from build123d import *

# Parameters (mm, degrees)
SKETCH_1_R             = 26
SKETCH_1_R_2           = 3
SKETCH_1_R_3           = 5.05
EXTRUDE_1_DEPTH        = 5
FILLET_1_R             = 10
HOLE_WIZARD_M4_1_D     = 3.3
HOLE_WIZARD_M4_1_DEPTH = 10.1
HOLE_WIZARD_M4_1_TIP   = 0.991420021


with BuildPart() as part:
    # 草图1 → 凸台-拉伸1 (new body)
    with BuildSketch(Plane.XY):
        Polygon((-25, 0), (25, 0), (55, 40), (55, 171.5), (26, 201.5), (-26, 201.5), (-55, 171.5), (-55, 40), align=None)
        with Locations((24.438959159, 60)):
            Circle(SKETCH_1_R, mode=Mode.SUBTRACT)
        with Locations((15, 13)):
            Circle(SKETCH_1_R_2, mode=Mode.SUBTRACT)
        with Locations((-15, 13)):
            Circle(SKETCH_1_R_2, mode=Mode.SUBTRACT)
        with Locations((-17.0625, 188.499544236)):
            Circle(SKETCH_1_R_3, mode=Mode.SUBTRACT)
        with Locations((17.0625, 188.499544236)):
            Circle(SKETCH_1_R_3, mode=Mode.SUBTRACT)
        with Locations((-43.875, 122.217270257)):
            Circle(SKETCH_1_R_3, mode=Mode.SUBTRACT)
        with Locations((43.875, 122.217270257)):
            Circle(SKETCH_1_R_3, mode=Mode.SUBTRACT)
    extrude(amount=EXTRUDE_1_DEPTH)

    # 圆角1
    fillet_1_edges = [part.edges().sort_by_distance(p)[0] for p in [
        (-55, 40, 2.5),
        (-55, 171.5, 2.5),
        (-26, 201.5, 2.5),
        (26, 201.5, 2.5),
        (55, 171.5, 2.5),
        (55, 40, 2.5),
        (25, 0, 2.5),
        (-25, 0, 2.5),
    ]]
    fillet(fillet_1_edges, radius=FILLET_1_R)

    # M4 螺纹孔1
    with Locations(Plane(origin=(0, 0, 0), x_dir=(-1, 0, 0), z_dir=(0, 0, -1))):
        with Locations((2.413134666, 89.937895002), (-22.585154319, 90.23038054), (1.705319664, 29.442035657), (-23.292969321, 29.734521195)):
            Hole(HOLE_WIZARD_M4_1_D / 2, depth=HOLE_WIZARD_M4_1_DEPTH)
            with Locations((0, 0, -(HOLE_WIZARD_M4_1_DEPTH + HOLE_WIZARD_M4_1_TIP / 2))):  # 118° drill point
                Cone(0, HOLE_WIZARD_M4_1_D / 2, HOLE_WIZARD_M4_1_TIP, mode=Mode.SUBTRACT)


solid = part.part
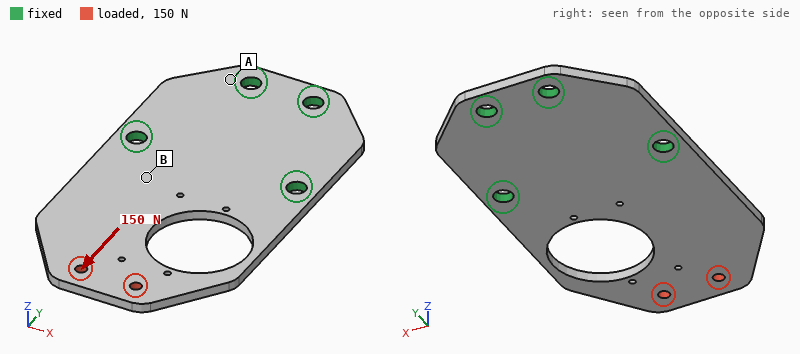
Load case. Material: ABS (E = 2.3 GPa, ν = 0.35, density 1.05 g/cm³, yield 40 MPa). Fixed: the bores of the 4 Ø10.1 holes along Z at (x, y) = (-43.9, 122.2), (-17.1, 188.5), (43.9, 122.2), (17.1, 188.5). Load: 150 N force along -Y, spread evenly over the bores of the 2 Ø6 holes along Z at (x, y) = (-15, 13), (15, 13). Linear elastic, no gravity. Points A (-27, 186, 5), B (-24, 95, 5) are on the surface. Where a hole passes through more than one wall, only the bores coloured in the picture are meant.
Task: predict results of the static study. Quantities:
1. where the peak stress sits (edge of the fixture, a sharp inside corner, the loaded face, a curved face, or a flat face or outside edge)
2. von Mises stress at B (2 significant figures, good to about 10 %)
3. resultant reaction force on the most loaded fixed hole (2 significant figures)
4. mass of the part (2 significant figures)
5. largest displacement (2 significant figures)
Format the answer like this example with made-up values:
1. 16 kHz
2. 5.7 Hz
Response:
1. a curved face
2. 0.46 MPa
3. 62 N
4. 92 g
5. 71 µm
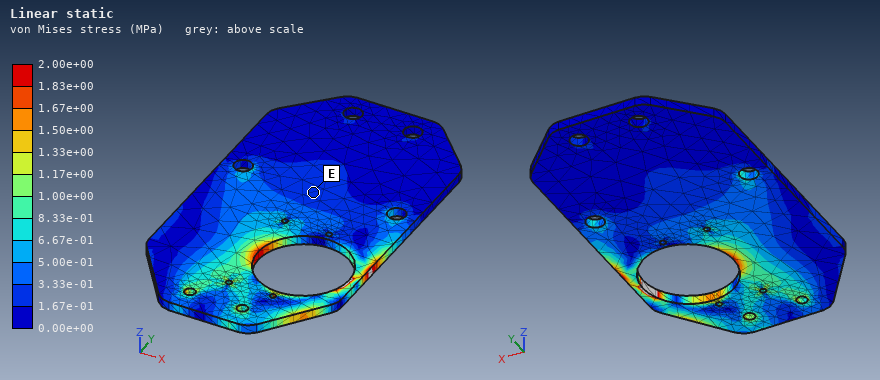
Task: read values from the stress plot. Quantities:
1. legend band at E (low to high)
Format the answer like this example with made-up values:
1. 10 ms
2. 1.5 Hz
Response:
1. 1.67e-01 to 3.33e-01 MPa
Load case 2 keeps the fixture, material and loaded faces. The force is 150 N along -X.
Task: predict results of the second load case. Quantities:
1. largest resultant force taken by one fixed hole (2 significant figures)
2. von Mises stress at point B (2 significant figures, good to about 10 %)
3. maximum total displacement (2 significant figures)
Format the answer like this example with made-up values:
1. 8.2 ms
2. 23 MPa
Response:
1. 200 N
2. 0.46 MPa
3. 0.22 mm
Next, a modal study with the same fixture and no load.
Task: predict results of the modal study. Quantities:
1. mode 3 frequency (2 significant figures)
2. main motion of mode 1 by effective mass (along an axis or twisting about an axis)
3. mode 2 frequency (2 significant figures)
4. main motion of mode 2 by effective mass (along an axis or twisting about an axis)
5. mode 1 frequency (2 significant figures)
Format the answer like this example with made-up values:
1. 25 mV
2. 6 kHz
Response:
1. 510 Hz
2. along Z
3. 270 Hz
4. twisting about Y
5. 89 Hz
